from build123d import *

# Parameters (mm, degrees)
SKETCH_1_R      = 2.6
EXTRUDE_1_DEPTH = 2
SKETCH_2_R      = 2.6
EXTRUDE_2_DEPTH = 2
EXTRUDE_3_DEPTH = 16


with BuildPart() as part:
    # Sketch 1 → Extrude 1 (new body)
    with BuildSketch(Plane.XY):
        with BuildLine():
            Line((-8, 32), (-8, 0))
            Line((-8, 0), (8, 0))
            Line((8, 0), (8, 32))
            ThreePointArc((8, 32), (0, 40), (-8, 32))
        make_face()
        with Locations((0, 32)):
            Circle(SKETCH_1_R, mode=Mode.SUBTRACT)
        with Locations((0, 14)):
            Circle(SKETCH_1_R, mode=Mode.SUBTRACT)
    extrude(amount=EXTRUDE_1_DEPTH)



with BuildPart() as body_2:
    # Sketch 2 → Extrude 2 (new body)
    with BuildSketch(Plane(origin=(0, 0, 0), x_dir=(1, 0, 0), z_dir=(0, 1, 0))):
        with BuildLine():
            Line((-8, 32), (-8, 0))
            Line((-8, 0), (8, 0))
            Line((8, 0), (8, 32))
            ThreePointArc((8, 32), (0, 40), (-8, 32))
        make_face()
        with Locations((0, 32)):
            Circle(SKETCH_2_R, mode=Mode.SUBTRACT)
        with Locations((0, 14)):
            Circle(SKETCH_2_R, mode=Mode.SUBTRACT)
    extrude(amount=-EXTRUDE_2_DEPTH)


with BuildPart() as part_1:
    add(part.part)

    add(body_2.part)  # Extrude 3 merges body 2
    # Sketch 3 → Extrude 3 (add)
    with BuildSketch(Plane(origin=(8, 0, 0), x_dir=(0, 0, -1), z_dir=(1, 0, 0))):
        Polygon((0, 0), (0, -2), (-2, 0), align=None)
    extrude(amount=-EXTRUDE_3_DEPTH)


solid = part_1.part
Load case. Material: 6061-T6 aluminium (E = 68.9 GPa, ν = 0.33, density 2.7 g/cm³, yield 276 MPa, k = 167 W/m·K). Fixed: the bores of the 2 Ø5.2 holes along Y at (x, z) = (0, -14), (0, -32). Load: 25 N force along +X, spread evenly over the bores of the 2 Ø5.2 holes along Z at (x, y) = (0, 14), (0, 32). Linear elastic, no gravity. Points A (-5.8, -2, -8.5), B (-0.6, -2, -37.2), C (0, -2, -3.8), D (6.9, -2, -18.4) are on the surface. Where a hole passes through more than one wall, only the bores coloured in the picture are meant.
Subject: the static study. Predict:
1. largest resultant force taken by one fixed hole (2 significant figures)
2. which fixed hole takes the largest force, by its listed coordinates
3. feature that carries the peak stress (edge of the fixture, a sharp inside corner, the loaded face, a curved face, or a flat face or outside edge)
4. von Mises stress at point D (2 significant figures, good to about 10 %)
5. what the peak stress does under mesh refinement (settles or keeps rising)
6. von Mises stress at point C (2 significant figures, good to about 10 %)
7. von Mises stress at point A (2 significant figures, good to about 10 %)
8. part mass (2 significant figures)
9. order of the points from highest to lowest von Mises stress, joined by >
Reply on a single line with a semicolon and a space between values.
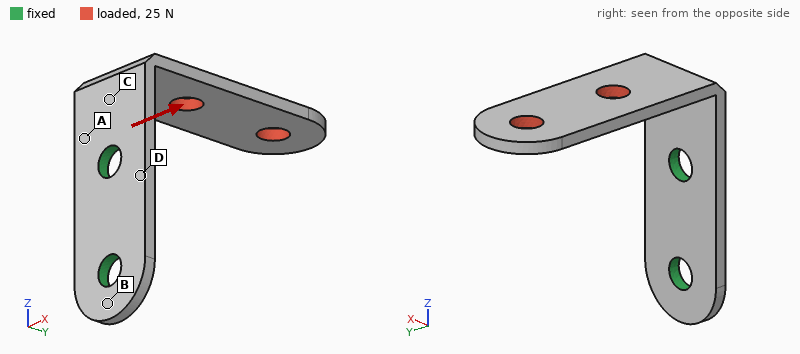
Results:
34 N; (0, -14); edge of the fixture; 10 MPa; keeps rising; 43 MPa; 34 MPa; 6.2 g; C > A > D > B
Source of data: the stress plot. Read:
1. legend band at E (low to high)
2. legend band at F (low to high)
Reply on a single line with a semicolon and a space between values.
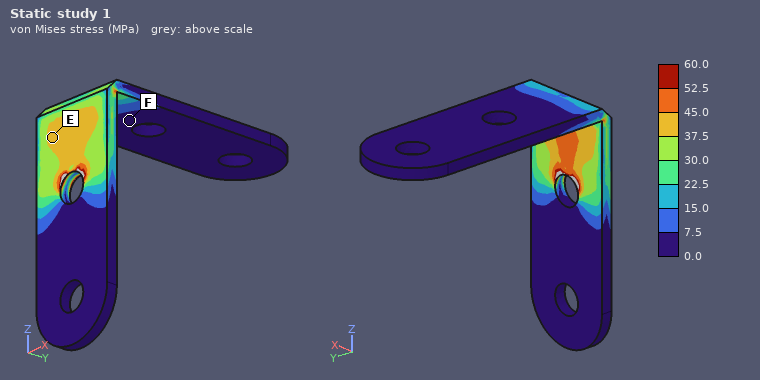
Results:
37.5 to 45.0 MPa; 0.0 to 7.5 MPa
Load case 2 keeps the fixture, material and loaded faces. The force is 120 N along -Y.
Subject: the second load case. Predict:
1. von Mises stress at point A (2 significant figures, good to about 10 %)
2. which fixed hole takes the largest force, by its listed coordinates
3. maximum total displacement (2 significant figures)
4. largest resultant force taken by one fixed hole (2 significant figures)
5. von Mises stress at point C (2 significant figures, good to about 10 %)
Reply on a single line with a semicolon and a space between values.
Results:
92 MPa; (0, -14); 0.60 mm; 120 N; 46 MPa
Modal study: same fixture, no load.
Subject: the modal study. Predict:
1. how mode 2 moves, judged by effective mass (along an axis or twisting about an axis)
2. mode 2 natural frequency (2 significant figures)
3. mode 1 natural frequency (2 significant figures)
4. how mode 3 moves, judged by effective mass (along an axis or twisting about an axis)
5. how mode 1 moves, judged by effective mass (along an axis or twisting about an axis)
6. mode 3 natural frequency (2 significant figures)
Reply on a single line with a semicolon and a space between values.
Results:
along X; 1200 Hz; 700 Hz; along Y; along Z; 3200 Hz
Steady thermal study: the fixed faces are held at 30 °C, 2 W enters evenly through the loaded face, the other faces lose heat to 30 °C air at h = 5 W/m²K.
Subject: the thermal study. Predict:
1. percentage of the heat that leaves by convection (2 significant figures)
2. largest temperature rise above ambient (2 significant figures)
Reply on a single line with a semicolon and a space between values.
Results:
4.1 %; 15 K
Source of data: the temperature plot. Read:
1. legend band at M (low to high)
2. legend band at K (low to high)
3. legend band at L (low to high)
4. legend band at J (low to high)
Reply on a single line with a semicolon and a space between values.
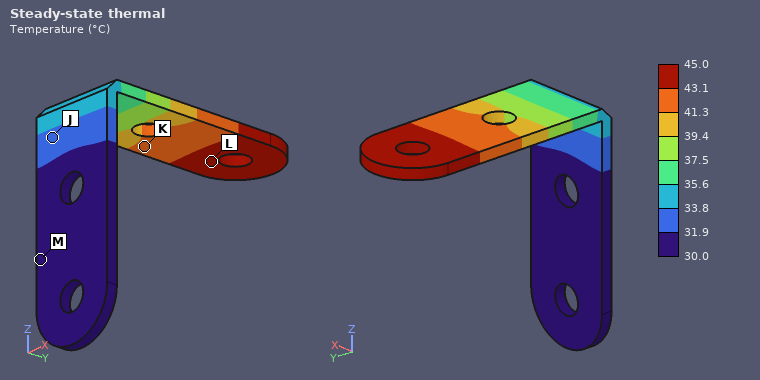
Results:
30.0 to 31.9 °C; 41.3 to 43.1 °C; 43.1 to 45.0 °C; 31.9 to 33.8 °C
